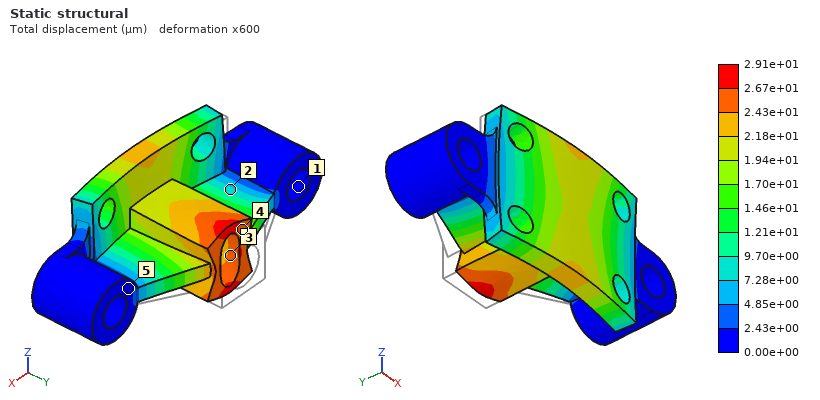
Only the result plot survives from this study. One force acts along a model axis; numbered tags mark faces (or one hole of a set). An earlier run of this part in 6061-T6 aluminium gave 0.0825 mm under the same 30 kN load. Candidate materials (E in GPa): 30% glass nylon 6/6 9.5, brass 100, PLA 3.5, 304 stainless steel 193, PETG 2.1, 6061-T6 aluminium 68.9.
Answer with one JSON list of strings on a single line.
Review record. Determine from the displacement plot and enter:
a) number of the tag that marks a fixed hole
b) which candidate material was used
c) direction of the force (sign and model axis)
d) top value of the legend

["1", "304 stainless steel", "-Y", "2.91e+01 µm"]
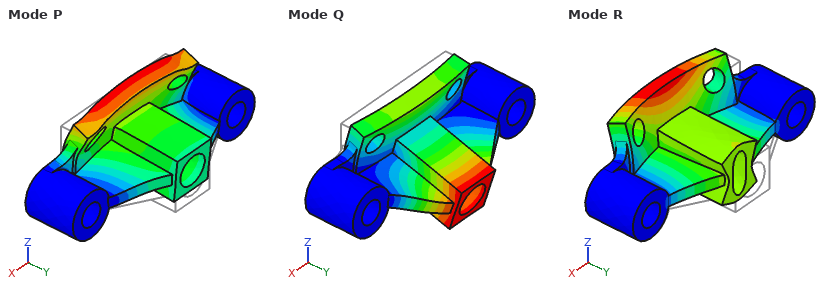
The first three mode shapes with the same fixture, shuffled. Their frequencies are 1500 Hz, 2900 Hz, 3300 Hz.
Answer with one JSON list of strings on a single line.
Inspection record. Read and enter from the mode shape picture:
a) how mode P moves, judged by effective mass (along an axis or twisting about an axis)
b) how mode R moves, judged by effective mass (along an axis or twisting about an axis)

["along Z", "along Y"]
